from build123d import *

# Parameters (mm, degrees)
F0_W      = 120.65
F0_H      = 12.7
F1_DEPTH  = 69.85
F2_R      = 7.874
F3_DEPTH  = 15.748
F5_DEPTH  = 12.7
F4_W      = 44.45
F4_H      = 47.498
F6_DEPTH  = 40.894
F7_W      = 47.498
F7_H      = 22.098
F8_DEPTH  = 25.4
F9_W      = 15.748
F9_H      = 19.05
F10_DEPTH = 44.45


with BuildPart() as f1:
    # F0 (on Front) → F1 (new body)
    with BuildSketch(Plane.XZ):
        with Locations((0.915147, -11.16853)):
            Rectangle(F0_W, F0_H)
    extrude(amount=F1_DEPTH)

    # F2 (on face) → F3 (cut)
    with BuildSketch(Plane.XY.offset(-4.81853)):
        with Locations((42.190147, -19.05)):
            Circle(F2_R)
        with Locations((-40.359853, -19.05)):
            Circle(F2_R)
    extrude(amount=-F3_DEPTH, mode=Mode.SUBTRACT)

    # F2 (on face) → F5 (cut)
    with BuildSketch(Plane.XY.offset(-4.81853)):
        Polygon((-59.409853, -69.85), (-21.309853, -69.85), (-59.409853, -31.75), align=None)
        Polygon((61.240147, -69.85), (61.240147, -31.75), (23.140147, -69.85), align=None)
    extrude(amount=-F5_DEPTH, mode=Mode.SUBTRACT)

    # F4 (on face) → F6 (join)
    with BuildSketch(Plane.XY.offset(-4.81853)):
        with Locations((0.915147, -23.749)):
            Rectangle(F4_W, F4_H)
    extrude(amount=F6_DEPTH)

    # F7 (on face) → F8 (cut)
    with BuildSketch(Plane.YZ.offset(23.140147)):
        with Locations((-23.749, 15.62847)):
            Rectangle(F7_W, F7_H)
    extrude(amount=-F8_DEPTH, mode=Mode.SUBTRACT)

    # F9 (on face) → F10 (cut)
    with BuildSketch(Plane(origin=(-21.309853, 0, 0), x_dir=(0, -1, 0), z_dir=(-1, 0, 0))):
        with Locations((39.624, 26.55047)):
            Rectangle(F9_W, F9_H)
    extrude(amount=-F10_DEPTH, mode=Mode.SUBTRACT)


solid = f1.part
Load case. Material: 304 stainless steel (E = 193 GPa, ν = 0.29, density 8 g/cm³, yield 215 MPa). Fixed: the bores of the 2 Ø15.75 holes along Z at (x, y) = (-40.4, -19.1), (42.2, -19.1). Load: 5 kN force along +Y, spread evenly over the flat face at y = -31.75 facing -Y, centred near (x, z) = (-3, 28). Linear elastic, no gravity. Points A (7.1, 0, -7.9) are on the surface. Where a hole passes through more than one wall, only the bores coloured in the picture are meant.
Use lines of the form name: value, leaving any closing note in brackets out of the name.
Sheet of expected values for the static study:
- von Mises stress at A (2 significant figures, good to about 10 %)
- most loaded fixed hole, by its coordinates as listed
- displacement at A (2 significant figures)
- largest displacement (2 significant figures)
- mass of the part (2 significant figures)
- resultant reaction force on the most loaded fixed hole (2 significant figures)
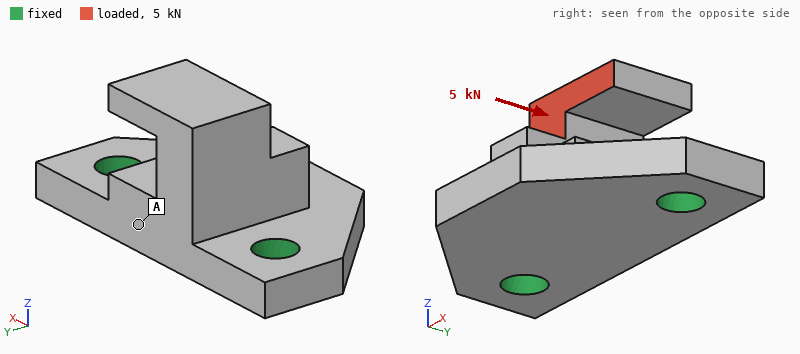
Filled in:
von Mises stress at A: 16 MPa
most loaded fixed hole, by its coordinates as listed: (-40.4, -19.1)
displacement at A: 13 µm
largest displacement: 56 µm
mass of the part: 1.1 kg
resultant reaction force on the most loaded fixed hole: 2.9 kN
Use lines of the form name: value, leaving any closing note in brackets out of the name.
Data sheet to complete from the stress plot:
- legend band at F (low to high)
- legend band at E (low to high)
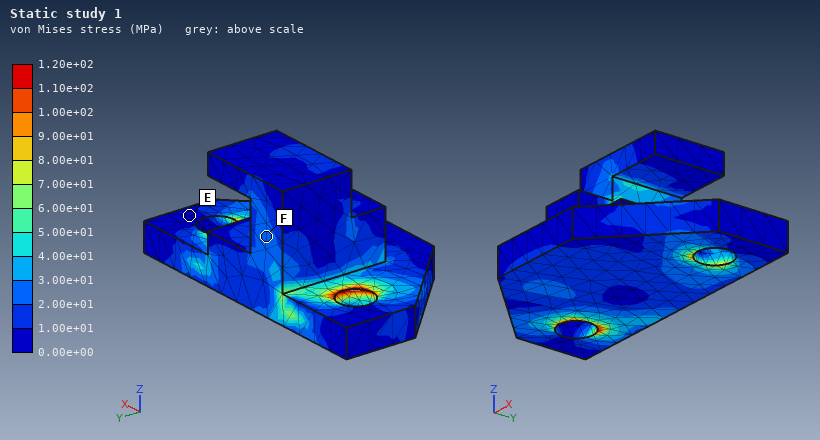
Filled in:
legend band at F: 2.00e+01 to 3.00e+01 MPa
legend band at E: 0.00e+00 to 1.00e+01 MPa
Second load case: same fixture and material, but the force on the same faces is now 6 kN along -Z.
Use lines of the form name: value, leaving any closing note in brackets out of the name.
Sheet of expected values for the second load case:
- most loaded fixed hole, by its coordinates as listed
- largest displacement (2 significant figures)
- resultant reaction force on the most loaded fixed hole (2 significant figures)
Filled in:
most loaded fixed hole, by its coordinates as listed: (-40.4, -19.1)
largest displacement: 69 µm
resultant reaction force on the most loaded fixed hole: 3.6 kN
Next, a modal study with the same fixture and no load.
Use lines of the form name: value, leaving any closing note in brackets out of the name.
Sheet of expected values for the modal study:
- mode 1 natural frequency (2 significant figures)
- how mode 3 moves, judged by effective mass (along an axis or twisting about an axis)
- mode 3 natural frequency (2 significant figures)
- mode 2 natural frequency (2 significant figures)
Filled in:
mode 1 natural frequency: 3300 Hz
how mode 3 moves, judged by effective mass: along Z
mode 3 natural frequency: 6600 Hz
mode 2 natural frequency: 4600 Hz
